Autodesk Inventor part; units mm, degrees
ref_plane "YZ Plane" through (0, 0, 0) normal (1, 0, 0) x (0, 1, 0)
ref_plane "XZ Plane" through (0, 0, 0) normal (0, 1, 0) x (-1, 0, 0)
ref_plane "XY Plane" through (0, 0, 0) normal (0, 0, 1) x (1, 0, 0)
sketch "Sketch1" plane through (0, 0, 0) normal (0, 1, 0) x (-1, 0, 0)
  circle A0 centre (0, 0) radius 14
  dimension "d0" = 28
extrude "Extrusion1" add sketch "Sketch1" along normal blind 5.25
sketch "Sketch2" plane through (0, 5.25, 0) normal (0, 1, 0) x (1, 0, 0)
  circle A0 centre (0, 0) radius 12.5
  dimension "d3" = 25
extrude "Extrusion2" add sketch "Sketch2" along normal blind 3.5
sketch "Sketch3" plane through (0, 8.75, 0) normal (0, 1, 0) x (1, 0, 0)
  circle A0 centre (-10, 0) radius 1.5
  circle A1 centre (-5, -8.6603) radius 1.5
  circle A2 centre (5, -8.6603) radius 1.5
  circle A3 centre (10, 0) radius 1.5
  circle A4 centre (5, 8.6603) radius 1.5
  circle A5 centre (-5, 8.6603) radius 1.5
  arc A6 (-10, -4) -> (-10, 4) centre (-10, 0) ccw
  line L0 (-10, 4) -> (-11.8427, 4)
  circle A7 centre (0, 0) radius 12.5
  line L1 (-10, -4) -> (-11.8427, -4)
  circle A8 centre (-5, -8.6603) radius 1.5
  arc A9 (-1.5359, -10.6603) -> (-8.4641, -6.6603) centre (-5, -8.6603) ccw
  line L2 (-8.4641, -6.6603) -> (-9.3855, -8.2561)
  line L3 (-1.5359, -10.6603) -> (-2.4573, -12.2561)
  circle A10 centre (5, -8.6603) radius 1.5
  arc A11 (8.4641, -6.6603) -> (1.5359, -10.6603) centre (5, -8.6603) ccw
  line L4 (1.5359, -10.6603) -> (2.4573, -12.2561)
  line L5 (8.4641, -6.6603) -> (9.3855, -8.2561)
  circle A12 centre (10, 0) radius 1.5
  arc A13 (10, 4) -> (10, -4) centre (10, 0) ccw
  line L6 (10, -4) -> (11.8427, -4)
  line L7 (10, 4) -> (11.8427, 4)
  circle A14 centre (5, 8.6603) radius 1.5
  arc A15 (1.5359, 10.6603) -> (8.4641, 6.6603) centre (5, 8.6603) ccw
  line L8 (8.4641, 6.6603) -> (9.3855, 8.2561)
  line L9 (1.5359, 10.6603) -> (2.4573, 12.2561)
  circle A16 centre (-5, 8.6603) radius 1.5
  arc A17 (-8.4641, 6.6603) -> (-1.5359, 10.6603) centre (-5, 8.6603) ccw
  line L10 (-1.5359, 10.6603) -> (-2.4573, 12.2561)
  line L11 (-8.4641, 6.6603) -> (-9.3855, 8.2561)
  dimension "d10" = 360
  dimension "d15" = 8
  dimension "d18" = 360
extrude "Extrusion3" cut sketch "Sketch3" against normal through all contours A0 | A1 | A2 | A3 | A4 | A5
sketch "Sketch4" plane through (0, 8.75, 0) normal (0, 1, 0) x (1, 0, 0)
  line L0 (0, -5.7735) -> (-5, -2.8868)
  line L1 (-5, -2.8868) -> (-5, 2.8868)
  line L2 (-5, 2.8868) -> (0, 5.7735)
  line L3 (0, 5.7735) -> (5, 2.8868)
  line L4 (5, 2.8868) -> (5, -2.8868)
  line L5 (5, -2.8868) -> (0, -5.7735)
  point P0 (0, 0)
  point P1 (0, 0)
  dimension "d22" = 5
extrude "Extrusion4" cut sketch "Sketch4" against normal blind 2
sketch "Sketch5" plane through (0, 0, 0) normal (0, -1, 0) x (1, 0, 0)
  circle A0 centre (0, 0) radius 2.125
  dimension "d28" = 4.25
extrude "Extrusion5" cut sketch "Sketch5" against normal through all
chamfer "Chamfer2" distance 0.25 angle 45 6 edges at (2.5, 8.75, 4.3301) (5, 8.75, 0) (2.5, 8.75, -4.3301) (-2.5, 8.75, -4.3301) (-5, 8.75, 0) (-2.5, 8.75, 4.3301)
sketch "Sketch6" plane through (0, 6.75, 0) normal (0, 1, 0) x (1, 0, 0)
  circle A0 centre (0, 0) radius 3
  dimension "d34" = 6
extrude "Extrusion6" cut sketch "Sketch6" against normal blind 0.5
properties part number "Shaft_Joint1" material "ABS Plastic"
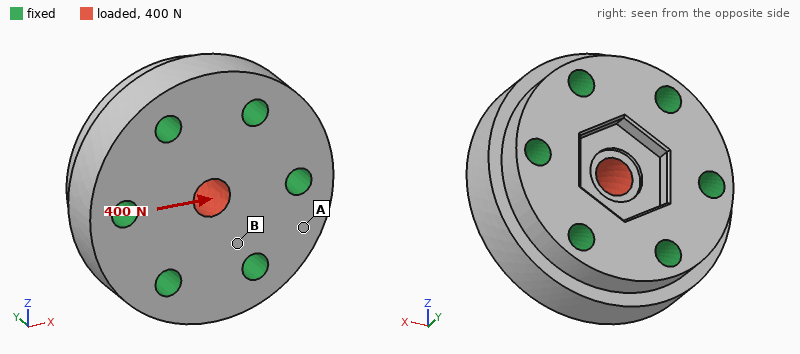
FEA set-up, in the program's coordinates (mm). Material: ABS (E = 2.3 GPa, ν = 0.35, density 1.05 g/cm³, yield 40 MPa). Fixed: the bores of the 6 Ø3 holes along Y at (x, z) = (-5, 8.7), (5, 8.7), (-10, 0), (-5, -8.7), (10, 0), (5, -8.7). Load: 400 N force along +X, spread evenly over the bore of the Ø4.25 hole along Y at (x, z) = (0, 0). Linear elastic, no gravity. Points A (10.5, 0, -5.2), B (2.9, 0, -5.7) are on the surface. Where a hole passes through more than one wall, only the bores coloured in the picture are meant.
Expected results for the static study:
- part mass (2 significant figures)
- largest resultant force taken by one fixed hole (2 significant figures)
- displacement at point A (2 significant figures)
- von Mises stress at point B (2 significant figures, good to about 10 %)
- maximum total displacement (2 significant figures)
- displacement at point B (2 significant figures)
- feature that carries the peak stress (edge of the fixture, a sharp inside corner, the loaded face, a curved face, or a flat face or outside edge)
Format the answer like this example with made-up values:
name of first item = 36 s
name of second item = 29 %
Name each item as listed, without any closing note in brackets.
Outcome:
part mass = 4.5 g
largest resultant force taken by one fixed hole = 110 N
displacement at point A = 2.0 µm
von Mises stress at point B = 1.7 MPa
maximum total displacement = 12 µm
displacement at point B = 2.1 µm
feature that carries the peak stress = a sharp inside corner
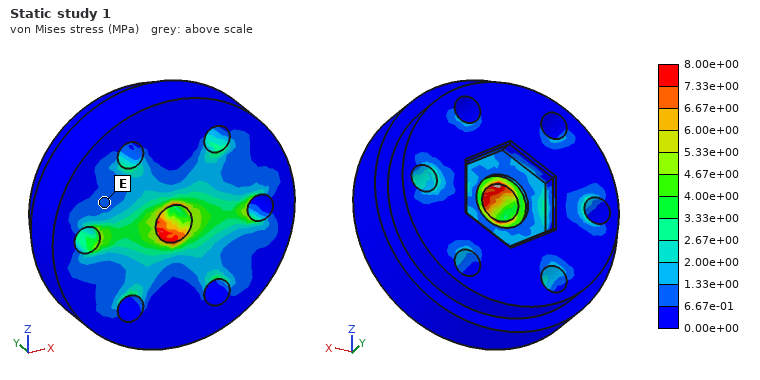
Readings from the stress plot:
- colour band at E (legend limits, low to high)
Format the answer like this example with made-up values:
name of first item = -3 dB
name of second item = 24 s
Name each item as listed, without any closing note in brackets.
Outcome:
colour band at E = 6.67e-01 to 1.33e+00 MPa
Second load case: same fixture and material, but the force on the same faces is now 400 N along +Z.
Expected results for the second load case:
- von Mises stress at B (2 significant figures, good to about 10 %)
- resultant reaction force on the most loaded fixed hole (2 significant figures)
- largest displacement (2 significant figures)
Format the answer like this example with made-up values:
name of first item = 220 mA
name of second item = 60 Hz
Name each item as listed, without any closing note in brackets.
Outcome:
von Mises stress at B = 3.1 MPa
resultant reaction force on the most loaded fixed hole = 98 N
largest displacement = 12 µm
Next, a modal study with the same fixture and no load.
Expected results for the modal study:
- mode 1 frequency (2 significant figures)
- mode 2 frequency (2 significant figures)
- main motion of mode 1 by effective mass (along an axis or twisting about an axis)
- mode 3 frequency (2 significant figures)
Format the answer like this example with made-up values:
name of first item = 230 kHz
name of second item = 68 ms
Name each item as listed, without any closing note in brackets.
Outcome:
mode 1 frequency = 32 kHz
mode 2 frequency = 39 kHz
main motion of mode 1 by effective mass = along Y
mode 3 frequency = 39 kHz
